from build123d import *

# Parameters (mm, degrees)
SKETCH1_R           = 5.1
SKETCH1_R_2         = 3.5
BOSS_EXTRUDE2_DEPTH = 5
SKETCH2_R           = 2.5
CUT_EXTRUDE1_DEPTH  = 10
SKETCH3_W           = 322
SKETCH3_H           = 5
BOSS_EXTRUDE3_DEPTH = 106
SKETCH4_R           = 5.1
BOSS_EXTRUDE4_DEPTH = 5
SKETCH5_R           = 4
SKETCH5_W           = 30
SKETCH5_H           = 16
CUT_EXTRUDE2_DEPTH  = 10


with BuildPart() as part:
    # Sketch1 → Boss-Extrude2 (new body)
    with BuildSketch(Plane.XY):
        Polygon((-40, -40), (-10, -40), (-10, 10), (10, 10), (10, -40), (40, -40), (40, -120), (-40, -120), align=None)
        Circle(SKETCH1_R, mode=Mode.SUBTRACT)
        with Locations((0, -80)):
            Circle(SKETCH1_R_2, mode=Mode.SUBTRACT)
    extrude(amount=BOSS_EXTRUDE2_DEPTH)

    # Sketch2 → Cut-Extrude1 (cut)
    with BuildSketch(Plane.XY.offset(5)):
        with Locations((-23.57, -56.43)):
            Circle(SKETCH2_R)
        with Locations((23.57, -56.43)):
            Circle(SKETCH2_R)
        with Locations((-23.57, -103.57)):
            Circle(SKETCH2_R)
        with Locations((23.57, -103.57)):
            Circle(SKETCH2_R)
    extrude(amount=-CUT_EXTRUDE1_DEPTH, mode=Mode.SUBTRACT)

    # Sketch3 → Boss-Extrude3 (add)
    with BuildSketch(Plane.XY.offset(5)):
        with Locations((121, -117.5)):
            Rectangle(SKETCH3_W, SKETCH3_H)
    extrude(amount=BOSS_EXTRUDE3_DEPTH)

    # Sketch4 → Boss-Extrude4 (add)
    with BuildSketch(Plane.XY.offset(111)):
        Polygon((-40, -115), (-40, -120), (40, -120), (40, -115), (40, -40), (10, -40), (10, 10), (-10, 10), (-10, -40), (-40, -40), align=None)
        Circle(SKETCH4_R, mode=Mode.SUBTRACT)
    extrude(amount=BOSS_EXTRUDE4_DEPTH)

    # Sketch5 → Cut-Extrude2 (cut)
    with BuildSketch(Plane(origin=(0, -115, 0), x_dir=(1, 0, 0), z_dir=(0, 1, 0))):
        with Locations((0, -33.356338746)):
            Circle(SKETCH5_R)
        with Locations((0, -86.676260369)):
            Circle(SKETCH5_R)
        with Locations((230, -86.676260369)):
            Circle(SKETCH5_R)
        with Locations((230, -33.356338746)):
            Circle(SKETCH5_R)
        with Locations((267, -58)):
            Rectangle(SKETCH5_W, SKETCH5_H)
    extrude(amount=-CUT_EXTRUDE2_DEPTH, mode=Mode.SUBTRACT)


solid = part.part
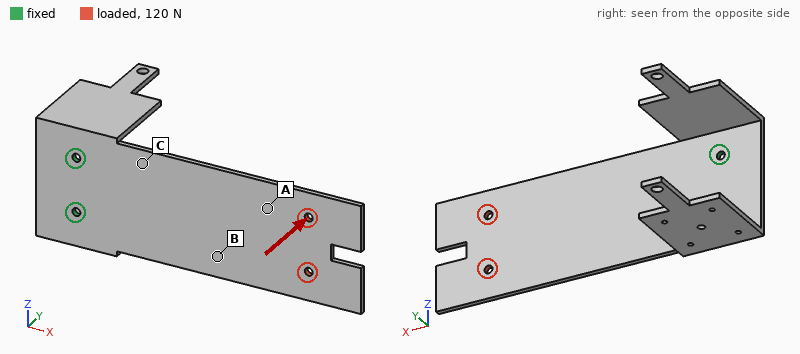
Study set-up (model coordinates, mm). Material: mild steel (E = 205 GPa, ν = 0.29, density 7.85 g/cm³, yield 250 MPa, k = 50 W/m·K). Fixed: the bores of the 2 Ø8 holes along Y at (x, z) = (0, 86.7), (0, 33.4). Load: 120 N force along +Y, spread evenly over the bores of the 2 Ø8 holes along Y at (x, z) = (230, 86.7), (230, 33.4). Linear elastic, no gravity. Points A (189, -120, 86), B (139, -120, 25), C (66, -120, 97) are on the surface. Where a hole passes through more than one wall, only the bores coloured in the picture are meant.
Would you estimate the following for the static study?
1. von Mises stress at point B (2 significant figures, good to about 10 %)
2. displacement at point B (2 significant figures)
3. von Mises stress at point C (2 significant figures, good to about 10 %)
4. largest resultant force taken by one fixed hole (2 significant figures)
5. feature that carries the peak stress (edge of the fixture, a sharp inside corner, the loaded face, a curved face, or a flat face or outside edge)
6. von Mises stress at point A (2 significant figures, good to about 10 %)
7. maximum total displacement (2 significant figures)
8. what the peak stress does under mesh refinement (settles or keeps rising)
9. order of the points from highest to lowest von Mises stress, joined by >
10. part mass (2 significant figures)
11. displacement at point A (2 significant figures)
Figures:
25 MPa
0.74 mm
46 MPa
84 N
edge of the fixture
12 MPa
2.4 mm
keeps rising
C > B > A
1.9 kg
1.3 mm
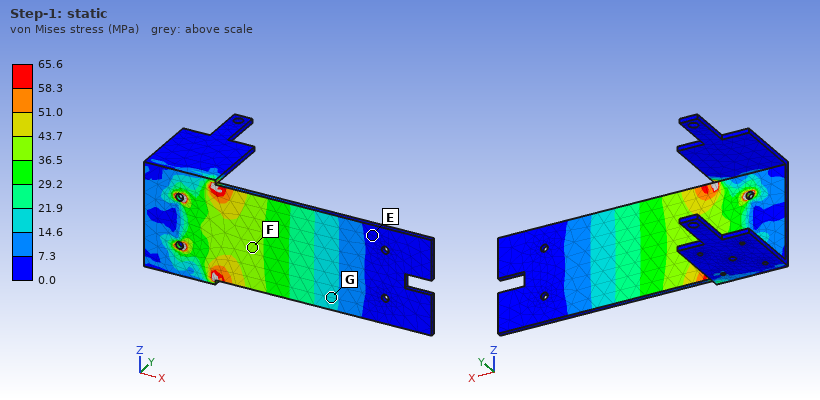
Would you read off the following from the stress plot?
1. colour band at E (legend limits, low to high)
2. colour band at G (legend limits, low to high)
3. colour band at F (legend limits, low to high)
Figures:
0.0 to 7.3 MPa
14.6 to 21.9 MPa
36.5 to 43.7 MPa
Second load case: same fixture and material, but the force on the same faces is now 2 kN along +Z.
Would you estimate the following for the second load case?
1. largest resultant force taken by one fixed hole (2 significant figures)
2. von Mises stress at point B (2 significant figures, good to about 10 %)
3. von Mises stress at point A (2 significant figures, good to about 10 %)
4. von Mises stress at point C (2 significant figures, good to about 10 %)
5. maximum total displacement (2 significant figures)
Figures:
8.1 kN
13 MPa
8.5 MPa
26 MPa
0.15 mm
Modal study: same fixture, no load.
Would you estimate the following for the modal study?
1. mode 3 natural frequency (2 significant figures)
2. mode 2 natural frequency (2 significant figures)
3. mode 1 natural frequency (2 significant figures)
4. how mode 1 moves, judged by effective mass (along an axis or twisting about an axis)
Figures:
310 Hz
290 Hz
59 Hz
along Y
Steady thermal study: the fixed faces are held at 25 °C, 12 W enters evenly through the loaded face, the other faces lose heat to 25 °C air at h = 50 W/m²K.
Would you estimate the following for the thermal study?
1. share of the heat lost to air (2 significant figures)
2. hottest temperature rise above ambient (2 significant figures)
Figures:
99 %
16 K
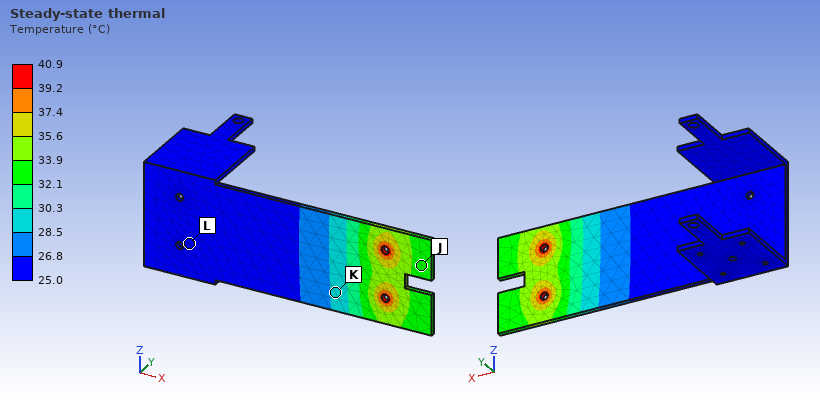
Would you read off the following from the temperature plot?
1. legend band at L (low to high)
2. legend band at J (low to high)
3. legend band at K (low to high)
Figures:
25.0 to 26.8 °C
32.1 to 33.9 °C
28.5 to 30.3 °C
